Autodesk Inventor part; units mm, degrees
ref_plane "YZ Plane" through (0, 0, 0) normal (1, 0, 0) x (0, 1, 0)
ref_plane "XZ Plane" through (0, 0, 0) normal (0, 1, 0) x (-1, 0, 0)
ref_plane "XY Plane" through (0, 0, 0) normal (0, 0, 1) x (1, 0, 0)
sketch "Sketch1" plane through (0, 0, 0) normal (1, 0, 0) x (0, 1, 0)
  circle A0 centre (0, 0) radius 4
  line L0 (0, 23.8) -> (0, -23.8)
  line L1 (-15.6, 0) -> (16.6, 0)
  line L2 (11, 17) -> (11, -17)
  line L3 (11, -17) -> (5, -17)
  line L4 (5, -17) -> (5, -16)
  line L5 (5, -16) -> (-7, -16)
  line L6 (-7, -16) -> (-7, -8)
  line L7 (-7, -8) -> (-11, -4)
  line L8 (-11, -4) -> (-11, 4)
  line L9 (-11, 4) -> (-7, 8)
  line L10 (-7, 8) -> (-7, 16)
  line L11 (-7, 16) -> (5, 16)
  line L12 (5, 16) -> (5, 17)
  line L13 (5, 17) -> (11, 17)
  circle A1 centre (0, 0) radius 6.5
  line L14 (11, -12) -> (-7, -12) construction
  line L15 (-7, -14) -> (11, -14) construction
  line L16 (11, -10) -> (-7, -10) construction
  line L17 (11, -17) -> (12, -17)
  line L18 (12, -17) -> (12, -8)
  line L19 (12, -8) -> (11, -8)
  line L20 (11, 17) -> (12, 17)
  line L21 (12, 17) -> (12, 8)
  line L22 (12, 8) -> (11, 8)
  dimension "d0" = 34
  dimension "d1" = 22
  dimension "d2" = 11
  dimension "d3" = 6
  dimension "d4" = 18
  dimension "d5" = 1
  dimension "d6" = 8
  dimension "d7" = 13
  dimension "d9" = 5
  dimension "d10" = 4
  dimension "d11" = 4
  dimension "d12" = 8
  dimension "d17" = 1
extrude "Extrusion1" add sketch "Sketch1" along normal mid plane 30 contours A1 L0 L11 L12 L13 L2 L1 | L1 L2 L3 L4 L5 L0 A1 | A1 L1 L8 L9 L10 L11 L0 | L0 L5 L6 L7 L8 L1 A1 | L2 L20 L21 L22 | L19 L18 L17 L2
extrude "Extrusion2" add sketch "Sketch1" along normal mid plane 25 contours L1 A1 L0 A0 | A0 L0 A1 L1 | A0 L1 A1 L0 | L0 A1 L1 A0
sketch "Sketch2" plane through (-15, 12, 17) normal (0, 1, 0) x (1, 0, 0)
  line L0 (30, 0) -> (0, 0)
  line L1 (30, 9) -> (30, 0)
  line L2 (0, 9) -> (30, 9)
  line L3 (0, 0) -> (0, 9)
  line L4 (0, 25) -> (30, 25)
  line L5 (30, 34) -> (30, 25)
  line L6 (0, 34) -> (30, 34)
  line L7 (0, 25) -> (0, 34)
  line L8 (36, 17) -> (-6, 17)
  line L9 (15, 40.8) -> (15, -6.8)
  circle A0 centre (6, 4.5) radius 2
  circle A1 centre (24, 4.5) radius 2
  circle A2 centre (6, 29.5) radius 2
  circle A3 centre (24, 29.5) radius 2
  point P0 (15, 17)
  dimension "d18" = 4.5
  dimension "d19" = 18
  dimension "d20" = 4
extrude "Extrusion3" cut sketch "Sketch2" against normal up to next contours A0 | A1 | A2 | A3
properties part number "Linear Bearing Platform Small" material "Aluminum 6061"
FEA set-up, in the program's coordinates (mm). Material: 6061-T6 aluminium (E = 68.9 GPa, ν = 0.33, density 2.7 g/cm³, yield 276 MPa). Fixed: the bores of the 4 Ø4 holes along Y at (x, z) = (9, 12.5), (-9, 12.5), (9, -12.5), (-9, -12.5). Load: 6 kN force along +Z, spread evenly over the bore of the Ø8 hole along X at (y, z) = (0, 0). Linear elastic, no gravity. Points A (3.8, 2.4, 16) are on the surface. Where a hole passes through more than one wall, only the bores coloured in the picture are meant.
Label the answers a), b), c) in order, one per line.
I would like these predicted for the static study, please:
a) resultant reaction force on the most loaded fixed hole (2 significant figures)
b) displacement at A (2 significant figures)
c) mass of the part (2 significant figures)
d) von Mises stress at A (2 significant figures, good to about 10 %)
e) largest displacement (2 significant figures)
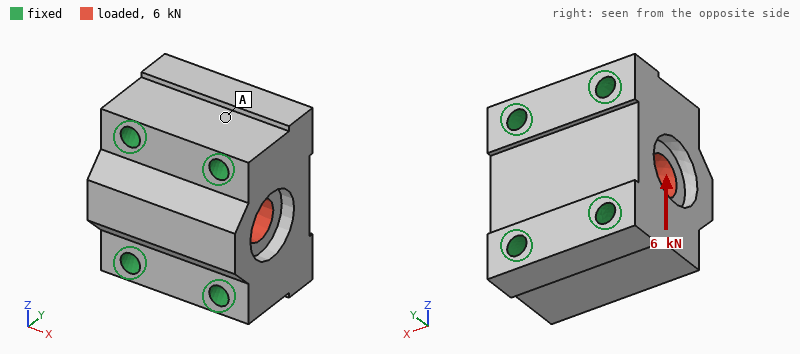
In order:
a) 1.5 kN
b) 0.57 µm
c) 45 g
d) 2.5 MPa
e) 1.9 µm
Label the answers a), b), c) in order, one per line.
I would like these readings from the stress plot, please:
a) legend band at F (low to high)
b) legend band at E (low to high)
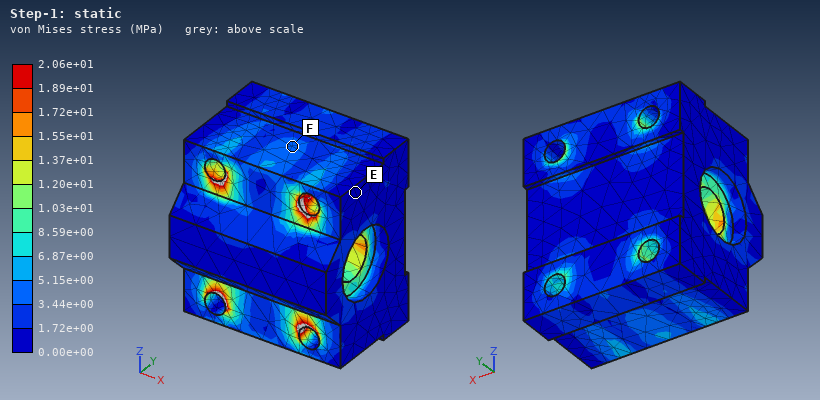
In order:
a) 3.44e+00 to 5.15e+00 MPa
b) 0.00e+00 to 1.72e+00 MPa
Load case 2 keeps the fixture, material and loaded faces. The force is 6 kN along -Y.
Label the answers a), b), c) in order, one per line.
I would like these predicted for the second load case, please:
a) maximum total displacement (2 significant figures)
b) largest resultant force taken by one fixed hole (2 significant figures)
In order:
a) 3.5 µm
b) 1.5 kN
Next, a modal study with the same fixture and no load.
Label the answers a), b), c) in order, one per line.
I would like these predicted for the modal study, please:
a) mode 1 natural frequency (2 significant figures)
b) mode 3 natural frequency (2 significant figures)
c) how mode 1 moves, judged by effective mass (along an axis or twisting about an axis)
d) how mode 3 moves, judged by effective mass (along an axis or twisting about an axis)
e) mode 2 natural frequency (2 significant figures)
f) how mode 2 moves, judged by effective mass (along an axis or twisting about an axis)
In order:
a) 51 kHz
b) 63 kHz
c) along X
d) along X
e) 55 kHz
f) along Y
